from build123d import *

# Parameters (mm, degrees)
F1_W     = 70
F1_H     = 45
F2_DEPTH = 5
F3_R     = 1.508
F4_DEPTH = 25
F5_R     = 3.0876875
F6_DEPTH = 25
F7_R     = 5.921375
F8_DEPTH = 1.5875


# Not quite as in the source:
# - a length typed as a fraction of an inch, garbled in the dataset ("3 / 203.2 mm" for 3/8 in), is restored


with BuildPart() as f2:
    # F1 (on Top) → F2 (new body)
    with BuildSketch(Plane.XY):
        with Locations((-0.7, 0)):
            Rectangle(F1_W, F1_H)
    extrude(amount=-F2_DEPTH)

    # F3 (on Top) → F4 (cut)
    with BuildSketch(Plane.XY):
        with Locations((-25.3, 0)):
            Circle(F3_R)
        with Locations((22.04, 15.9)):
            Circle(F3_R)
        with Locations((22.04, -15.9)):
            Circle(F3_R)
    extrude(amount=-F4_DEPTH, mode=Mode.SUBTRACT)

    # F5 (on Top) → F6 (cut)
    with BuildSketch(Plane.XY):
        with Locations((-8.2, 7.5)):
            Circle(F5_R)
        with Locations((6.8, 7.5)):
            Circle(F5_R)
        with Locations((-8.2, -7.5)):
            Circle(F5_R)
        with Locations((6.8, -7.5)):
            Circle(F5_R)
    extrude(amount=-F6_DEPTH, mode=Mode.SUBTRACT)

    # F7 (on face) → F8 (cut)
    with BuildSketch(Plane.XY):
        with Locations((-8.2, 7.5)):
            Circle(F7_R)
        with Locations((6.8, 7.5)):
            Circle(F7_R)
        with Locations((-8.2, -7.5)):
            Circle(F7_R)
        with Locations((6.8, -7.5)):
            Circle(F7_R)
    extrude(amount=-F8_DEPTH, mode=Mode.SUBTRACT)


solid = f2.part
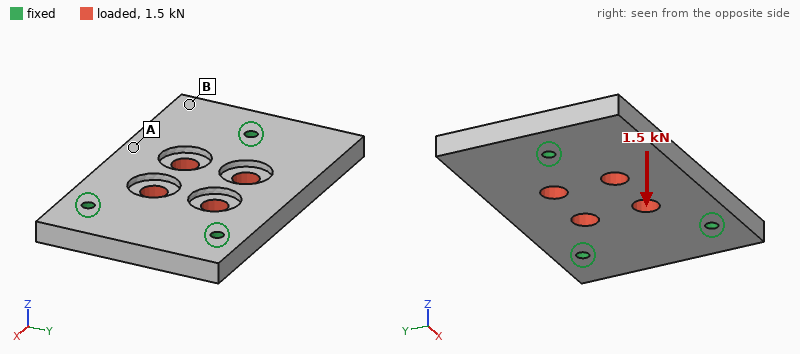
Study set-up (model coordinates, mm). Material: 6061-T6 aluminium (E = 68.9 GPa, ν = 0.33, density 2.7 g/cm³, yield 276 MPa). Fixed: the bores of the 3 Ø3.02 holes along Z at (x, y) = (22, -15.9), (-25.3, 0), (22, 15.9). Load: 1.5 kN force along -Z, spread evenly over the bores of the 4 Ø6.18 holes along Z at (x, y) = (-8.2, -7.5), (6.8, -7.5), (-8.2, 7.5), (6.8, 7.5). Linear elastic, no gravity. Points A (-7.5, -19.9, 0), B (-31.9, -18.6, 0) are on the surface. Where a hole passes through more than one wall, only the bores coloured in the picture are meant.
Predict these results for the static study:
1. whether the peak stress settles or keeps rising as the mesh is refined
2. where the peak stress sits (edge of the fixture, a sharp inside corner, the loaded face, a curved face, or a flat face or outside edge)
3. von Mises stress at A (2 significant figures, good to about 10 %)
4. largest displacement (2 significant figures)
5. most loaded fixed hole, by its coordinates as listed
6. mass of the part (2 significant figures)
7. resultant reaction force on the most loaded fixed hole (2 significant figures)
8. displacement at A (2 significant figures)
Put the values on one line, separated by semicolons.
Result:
keeps rising; edge of the fixture; 32 MPa; 47 µm; (-25.3, 0); 39 g; 700 N; 32 µm
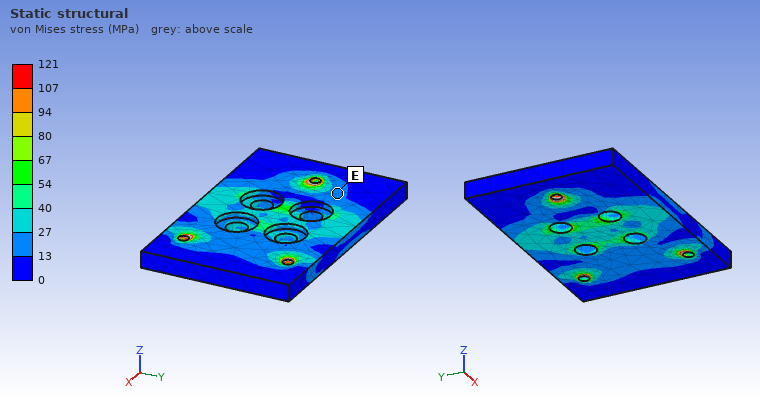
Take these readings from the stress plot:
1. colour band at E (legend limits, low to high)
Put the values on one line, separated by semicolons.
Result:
13 to 27 MPa
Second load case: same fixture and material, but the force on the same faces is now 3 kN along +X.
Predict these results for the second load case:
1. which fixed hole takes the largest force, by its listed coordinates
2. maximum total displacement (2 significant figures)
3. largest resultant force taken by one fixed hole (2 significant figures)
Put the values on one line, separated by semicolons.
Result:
(-25.3, 0); 5.3 µm; 1.2 kN
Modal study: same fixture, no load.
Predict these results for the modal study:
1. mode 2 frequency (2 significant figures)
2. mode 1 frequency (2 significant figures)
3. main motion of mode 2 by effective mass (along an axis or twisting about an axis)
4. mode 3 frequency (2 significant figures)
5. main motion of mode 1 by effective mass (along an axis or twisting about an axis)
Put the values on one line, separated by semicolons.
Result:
7500 Hz; 6200 Hz; along Z; 10 kHz; twisting about X
